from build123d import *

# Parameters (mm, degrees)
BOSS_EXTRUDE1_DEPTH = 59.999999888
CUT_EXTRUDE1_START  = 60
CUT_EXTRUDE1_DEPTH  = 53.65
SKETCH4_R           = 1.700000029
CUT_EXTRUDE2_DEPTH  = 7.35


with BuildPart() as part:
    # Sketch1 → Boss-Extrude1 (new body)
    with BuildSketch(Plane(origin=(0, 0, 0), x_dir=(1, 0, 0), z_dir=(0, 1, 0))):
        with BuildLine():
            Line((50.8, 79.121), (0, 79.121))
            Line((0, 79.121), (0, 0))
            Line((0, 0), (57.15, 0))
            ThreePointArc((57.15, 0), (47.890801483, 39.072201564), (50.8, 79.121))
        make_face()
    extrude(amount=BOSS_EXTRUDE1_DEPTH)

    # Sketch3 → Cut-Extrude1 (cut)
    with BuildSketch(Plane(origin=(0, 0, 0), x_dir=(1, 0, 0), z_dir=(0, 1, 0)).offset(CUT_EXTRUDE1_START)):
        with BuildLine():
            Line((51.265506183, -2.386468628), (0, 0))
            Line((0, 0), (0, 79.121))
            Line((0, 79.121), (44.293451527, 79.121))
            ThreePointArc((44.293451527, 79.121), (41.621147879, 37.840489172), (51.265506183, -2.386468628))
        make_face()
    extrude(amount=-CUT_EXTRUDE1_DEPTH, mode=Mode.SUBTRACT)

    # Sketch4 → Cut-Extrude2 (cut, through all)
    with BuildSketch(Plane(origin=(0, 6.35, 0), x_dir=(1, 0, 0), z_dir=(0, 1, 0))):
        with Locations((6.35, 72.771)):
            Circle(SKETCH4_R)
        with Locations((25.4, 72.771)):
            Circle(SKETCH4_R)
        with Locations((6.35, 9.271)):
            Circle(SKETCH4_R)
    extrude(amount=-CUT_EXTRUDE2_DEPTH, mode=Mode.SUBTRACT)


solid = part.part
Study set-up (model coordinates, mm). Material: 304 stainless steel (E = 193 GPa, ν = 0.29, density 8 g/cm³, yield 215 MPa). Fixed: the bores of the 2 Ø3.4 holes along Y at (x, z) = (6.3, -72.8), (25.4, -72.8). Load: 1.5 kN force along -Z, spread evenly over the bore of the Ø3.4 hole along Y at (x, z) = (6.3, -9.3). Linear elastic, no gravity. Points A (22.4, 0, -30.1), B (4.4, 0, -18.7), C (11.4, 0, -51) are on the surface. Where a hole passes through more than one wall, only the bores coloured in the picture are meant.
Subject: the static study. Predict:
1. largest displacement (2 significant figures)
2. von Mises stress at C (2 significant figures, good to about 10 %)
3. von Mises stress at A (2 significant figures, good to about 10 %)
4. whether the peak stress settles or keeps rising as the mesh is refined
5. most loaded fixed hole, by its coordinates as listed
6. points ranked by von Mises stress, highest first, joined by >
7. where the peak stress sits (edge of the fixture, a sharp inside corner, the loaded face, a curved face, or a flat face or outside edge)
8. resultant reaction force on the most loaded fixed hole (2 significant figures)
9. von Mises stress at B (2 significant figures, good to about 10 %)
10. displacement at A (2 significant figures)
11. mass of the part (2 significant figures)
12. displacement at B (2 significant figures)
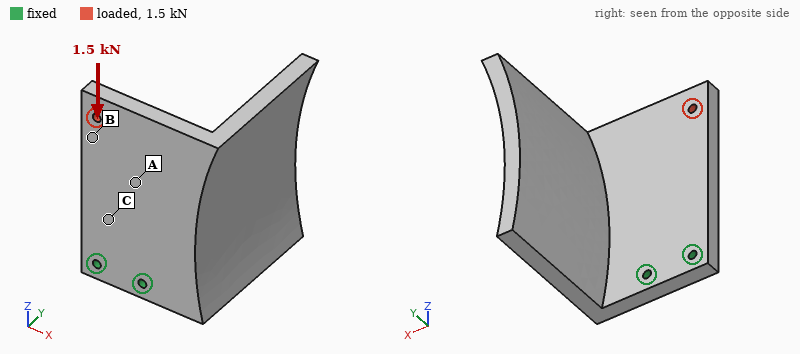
10 µm
10 MPa
4.1 MPa
keeps rising
(6.3, -72.8)
B > C > A
edge of the fixture
1.4 kN
16 MPa
3.7 µm
420 g
6.9 µm
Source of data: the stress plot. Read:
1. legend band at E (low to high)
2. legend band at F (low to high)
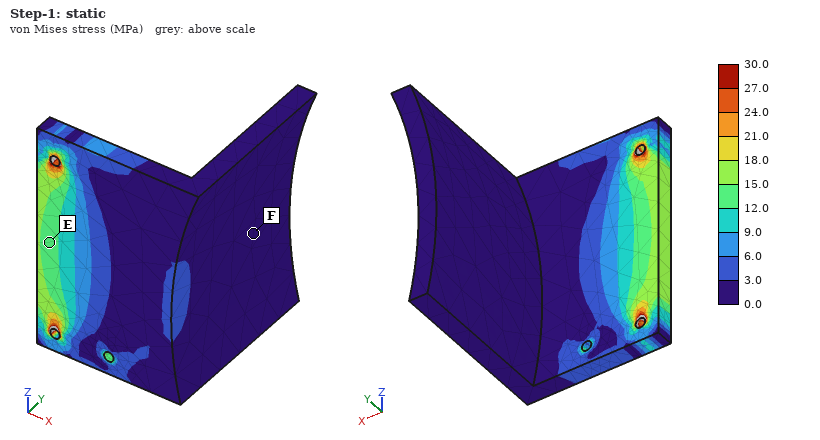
12.0 to 15.0 MPa
0.0 to 3.0 MPa
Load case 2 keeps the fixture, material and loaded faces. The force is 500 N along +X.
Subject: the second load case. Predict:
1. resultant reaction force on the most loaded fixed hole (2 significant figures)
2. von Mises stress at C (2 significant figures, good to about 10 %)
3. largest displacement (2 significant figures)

1.5 kN
7.7 MPa
15 µm
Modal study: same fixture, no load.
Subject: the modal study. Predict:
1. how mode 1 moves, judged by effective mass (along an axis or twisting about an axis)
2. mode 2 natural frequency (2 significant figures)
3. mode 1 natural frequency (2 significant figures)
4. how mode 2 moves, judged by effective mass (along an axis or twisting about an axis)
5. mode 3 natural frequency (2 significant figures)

along Y
830 Hz
500 Hz
along X
2200 Hz
